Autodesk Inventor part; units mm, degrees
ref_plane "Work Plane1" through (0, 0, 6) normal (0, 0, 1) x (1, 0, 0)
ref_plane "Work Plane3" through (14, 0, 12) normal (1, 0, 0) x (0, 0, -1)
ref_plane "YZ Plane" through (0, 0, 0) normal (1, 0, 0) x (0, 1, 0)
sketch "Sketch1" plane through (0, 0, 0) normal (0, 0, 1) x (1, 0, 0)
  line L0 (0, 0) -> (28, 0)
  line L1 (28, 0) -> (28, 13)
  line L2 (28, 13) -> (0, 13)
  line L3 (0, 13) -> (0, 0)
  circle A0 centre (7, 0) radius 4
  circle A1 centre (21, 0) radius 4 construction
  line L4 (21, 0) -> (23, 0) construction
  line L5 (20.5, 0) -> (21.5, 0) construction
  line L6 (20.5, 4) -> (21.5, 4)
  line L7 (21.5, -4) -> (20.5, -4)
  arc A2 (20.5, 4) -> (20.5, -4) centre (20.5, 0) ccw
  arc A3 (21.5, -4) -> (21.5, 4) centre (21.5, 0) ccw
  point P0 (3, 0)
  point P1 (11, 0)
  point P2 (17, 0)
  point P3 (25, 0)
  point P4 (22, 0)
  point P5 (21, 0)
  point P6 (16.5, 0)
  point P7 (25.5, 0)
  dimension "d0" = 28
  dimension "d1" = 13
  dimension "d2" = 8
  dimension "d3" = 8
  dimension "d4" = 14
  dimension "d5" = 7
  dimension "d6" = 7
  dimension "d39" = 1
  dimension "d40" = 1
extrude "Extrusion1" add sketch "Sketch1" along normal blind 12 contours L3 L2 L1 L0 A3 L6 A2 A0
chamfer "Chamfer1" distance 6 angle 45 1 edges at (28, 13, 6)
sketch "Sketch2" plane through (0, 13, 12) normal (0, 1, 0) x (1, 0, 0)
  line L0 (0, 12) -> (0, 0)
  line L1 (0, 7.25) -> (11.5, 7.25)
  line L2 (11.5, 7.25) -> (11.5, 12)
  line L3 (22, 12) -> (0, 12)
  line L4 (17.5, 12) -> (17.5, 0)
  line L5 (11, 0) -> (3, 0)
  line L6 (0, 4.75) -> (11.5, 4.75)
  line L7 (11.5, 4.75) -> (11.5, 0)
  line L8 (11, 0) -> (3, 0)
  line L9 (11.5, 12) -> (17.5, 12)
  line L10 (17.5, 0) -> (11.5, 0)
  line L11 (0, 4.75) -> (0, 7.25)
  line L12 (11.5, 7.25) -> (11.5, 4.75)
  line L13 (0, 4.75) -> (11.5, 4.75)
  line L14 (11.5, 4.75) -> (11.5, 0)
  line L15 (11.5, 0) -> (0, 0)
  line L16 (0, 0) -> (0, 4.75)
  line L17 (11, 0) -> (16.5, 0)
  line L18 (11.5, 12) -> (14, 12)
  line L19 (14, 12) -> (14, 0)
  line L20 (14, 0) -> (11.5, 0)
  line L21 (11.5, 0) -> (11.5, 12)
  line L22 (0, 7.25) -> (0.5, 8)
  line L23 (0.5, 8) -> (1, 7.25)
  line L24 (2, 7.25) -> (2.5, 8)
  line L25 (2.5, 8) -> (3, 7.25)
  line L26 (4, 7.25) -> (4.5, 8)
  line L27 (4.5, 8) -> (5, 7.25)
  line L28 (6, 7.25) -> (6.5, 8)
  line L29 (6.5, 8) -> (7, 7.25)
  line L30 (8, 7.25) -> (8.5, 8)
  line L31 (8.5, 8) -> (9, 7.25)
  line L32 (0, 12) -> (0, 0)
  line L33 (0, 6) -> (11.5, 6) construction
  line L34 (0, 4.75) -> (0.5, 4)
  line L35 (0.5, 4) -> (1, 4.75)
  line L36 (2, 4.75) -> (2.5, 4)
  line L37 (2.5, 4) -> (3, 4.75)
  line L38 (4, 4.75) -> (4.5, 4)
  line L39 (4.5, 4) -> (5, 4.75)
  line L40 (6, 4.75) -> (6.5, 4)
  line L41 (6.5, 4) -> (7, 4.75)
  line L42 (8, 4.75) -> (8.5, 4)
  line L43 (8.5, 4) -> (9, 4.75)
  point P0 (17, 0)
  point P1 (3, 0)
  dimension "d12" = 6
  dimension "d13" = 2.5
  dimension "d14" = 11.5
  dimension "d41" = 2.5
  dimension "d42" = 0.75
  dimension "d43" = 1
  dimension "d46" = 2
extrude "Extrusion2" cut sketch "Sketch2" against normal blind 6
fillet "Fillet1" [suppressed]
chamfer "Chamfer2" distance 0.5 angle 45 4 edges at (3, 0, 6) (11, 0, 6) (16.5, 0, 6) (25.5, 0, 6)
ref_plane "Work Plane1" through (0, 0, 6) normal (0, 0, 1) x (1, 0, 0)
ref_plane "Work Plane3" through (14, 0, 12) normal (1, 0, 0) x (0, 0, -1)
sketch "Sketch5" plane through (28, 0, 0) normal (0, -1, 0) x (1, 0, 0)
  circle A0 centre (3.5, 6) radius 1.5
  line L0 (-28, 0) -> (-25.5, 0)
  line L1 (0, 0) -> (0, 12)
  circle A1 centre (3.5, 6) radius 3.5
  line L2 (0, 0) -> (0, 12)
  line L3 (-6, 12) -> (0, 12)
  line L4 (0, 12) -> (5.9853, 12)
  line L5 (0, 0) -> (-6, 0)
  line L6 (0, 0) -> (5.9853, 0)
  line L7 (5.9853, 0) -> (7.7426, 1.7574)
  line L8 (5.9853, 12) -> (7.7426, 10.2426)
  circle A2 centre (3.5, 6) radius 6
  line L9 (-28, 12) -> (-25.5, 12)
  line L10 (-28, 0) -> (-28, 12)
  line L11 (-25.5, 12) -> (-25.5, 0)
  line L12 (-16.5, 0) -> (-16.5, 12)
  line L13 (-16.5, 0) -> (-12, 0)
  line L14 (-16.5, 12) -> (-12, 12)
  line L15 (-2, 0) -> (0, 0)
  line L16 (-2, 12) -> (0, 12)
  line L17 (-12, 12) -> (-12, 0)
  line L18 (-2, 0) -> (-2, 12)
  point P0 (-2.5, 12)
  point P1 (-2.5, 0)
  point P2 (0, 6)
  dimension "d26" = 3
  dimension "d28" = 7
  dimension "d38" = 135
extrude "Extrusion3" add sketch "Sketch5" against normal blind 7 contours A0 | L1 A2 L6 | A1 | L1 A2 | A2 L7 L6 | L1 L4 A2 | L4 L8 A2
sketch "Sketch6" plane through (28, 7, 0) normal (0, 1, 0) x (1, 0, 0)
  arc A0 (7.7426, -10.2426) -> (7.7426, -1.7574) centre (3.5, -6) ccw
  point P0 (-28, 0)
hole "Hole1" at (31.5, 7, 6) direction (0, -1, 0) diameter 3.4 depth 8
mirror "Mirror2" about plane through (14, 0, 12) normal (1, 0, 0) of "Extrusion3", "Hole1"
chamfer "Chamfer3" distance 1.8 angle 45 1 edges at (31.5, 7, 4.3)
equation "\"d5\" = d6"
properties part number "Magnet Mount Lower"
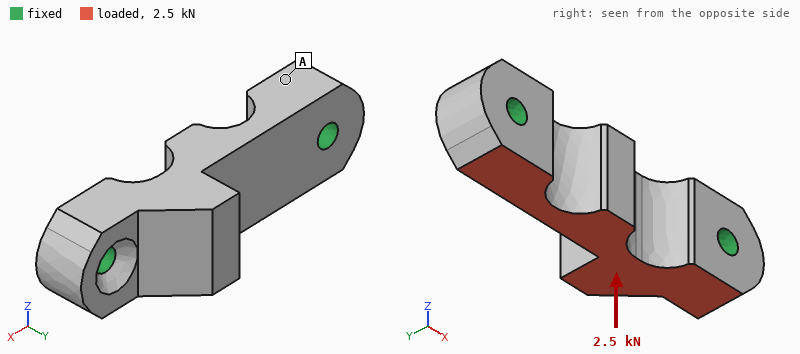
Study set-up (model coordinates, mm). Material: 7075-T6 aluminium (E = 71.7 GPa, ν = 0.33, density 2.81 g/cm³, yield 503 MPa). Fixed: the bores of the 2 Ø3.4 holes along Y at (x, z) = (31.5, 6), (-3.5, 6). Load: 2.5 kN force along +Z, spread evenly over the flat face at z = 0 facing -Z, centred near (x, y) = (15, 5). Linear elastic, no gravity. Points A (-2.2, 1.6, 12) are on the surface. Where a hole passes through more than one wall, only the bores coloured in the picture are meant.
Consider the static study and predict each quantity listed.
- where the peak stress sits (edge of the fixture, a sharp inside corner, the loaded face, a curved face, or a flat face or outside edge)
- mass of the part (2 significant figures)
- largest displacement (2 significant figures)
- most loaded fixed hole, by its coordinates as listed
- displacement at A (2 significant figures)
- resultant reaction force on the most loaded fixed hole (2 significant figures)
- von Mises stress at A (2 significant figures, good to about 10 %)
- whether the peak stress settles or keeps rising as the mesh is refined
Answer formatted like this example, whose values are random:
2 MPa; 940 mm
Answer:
edge of the fixture; 9.8 g; 26 µm; (31.5, 6); 4.2 µm; 1.3 kN; 18 MPa; keeps rising
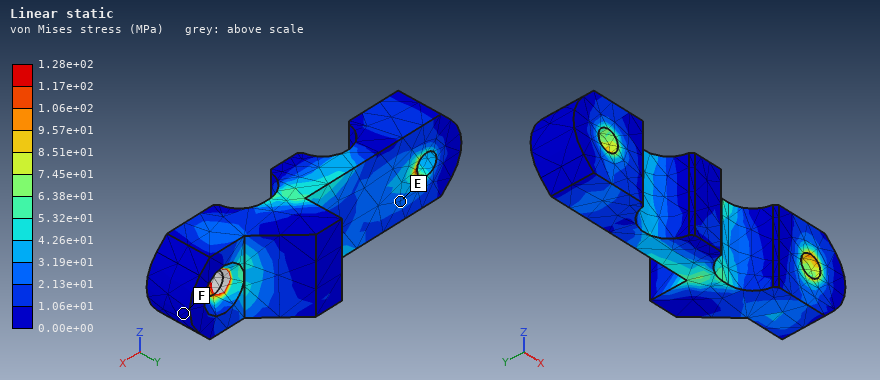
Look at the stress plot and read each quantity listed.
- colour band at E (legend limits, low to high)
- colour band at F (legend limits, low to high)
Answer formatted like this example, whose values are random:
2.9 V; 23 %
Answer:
2.13e+01 to 3.19e+01 MPa; 0.00e+00 to 1.06e+01 MPa
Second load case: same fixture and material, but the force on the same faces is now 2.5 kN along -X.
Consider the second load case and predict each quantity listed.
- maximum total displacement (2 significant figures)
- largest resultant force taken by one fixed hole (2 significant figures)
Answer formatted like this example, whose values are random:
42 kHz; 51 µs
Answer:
14 µm; 1.3 kN
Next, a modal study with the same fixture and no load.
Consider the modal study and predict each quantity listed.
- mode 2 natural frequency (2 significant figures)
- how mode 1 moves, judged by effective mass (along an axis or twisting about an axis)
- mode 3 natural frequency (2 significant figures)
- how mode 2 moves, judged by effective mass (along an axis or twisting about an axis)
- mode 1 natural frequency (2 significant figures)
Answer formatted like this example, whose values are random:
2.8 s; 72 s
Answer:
21 kHz; along Y; 25 kHz; along Z; 18 kHz
